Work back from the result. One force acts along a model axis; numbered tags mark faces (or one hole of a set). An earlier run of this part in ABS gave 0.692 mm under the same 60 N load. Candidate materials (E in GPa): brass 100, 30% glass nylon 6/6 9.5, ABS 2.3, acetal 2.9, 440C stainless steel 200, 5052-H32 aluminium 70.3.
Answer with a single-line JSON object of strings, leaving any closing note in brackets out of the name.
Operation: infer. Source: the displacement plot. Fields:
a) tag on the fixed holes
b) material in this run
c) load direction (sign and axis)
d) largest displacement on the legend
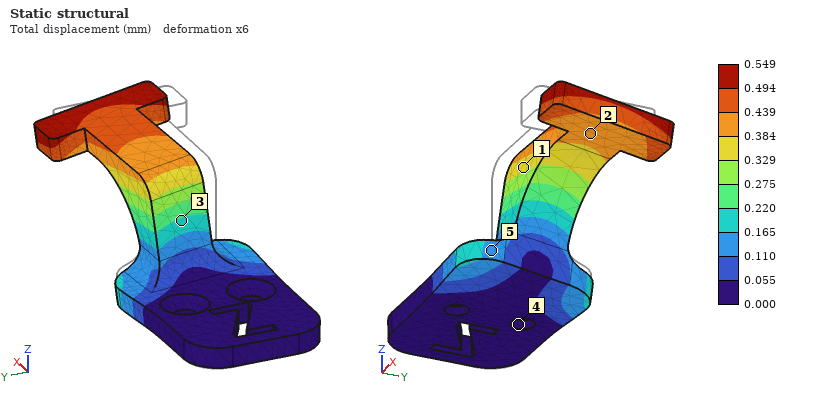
{"tag on the fixed holes": "4", "material in this run": "acetal", "load direction": "+Y", "largest displacement on the legend": "0.549 mm"}
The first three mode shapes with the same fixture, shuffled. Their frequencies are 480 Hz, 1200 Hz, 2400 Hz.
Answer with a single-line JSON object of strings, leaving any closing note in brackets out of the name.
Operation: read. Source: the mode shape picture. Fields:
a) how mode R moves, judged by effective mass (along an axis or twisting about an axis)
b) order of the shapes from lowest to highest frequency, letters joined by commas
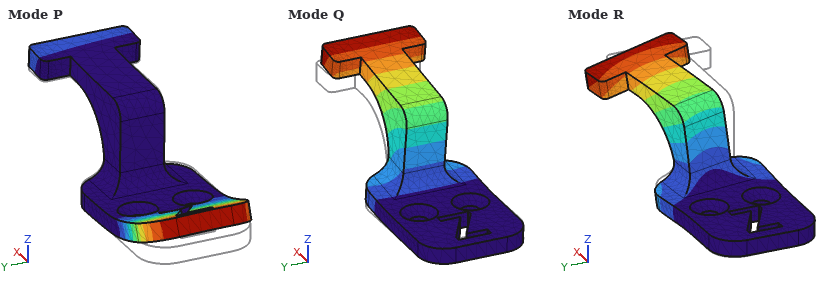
{"how mode R moves, judged by effective mass": "along Y", "order of the shapes from lowest to highest frequency, letters joined by commas": "Q, R, P"}
